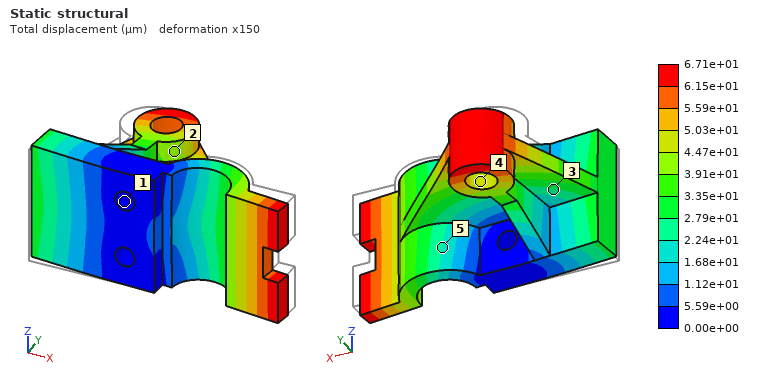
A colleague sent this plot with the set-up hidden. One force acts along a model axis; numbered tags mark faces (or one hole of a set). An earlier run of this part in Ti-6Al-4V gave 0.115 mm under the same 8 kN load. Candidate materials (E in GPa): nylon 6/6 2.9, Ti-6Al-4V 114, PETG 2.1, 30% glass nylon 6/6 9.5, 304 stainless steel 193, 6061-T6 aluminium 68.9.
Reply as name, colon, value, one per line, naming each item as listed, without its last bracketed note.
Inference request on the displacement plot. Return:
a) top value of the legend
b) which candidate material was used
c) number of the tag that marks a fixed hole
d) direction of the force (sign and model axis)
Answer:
top value of the legend: 6.71e+01 µm
which candidate material was used: 304 stainless steel
number of the tag that marks a fixed hole: 1
direction of the force: +X
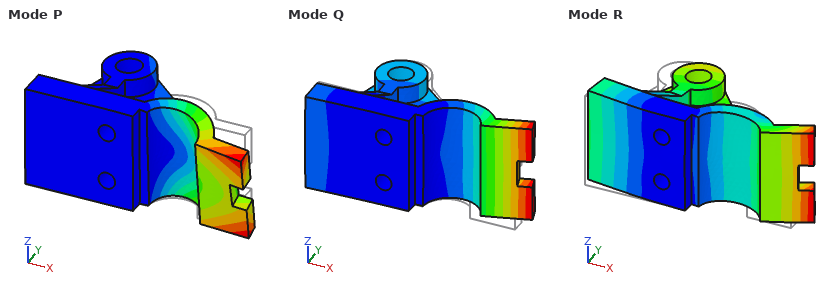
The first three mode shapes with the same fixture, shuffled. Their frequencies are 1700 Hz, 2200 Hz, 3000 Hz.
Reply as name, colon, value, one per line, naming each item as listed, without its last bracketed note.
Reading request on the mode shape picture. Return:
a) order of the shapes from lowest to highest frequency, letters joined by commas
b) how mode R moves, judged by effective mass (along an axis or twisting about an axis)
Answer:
order of the shapes from lowest to highest frequency, letters joined by commas: Q, P, R
how mode R moves, judged by effective mass: along X
